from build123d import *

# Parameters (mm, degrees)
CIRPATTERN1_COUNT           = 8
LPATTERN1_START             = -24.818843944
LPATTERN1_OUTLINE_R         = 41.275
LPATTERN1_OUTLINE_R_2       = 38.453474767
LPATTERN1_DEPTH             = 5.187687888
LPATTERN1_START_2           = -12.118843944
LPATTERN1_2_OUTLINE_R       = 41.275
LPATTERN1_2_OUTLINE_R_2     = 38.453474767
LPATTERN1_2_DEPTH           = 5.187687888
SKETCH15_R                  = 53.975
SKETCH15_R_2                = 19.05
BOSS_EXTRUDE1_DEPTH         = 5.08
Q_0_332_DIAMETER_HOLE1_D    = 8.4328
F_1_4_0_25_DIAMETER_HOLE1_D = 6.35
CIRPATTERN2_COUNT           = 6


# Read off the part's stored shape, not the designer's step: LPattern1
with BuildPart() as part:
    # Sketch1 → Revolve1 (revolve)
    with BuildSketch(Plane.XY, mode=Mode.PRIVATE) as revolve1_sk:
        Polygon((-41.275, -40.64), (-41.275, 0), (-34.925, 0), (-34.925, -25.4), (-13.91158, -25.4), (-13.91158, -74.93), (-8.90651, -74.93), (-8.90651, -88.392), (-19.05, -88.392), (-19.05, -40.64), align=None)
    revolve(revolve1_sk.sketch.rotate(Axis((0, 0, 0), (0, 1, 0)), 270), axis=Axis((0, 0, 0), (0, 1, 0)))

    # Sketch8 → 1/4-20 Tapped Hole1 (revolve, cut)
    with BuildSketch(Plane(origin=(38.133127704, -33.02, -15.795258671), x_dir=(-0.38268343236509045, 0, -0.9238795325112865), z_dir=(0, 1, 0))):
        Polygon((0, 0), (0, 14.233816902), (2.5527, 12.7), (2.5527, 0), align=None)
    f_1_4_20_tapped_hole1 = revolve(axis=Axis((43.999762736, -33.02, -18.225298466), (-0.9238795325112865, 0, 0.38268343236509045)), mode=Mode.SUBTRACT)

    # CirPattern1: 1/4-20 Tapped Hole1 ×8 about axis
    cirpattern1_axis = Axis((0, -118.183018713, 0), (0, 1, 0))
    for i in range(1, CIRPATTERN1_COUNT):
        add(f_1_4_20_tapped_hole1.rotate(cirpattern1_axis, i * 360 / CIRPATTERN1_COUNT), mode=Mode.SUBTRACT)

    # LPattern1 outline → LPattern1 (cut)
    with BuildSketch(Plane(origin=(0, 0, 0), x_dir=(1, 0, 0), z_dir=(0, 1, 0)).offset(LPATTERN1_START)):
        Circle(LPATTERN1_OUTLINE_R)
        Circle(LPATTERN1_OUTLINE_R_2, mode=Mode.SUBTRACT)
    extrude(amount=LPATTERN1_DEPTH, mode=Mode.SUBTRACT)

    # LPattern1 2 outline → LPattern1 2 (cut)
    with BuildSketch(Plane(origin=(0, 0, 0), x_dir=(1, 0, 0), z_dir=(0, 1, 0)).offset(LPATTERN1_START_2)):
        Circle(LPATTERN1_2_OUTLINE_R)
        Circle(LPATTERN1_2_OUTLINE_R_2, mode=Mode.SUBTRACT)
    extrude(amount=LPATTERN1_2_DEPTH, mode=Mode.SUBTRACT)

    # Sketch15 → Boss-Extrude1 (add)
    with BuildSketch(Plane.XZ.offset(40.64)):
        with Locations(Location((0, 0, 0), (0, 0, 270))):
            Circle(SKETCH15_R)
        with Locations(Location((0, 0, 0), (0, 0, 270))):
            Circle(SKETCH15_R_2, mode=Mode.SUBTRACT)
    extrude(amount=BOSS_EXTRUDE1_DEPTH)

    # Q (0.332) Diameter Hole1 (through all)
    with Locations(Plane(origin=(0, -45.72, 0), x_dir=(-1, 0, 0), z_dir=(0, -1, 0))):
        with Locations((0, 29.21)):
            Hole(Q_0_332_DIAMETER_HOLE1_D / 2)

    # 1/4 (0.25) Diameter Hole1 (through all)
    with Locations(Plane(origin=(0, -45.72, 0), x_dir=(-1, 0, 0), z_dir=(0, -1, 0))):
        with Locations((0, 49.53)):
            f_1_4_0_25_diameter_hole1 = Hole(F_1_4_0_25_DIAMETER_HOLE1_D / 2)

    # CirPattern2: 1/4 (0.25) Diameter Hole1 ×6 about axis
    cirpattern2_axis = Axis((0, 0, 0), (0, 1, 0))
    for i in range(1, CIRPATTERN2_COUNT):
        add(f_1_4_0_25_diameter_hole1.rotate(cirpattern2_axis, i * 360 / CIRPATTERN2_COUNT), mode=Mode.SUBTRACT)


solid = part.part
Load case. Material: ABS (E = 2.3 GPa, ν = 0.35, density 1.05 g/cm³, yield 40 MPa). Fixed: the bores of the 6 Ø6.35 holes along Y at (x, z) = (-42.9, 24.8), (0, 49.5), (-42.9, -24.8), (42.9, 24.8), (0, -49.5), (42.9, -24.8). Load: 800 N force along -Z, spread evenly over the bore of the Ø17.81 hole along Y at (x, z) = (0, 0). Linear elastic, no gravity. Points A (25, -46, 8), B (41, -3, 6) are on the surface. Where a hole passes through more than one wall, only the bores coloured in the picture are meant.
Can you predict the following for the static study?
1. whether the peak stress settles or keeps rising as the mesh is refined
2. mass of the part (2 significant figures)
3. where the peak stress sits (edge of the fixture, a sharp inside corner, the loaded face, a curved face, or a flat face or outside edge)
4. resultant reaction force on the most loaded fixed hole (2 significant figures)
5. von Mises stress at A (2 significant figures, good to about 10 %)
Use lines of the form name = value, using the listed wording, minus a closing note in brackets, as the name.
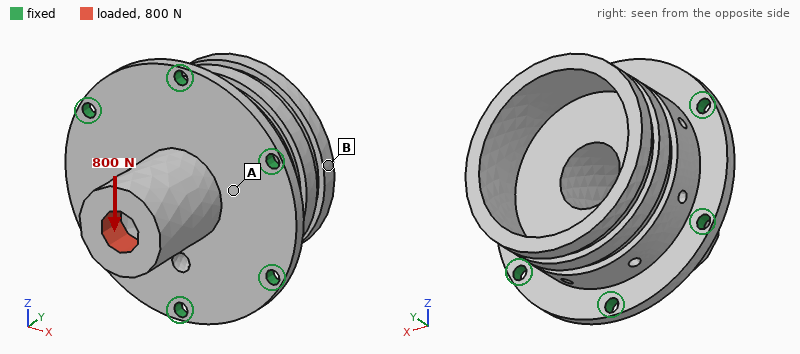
whether the peak stress settles or keeps rising as the mesh is refined = keeps rising
mass of the part = 180 g
where the peak stress sits = edge of the fixture
resultant reaction force on the most loaded fixed hole = 250 N
von Mises stress at A = 2.2 MPa
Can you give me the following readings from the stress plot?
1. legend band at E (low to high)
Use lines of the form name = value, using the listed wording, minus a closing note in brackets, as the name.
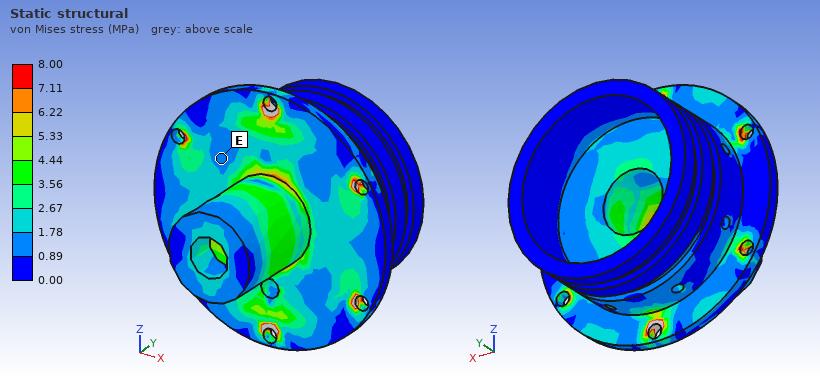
legend band at E = 0.89 to 1.78 MPa
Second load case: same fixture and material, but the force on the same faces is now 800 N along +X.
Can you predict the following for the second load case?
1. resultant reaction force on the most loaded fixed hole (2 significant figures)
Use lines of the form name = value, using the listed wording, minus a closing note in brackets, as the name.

resultant reaction force on the most loaded fixed hole = 230 N
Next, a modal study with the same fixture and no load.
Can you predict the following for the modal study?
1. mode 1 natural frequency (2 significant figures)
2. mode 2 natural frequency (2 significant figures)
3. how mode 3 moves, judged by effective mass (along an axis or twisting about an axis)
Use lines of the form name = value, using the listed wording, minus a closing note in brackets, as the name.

mode 1 natural frequency = 1600 Hz
mode 2 natural frequency = 1600 Hz
how mode 3 moves, judged by effective mass = along Y
